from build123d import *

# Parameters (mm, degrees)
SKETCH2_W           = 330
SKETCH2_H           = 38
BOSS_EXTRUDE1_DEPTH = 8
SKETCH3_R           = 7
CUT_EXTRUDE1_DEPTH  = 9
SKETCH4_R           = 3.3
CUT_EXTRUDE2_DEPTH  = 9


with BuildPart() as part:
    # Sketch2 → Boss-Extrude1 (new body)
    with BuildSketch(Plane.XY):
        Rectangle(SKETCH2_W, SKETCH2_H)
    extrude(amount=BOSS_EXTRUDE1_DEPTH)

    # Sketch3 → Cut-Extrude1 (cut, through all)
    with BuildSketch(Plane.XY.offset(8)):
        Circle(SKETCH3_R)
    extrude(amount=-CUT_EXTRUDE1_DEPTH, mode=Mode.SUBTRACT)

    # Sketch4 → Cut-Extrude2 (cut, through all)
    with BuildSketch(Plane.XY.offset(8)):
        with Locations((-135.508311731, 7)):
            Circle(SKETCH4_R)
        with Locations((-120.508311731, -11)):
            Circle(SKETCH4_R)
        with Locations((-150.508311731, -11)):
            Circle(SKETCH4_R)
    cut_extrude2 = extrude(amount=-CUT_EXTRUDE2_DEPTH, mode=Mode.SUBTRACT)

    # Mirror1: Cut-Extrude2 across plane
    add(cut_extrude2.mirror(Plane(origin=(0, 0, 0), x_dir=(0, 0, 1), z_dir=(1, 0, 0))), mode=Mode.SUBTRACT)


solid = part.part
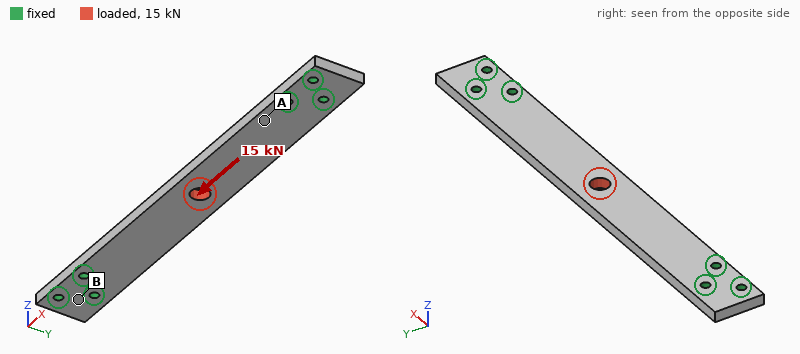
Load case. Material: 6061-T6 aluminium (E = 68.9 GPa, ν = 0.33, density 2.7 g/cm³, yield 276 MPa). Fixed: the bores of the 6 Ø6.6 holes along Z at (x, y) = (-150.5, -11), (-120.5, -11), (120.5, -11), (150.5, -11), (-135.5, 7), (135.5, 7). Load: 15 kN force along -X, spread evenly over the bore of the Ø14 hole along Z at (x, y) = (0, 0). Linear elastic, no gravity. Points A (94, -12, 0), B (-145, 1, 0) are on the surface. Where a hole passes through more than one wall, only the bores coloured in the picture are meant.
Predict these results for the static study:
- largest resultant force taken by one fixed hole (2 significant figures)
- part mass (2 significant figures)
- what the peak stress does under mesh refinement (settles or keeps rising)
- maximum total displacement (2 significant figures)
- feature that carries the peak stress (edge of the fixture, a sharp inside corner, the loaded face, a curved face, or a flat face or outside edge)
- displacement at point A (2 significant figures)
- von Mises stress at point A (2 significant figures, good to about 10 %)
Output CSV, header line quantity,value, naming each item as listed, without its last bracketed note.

quantity,value
largest resultant force taken by one fixed hole,4.1 kN
part mass,260 g
what the peak stress does under mesh refinement,keeps rising
maximum total displacement,49 µm
feature that carries the peak stress,edge of the fixture
displacement at point A,11 µm
von Mises stress at point A,28 MPa
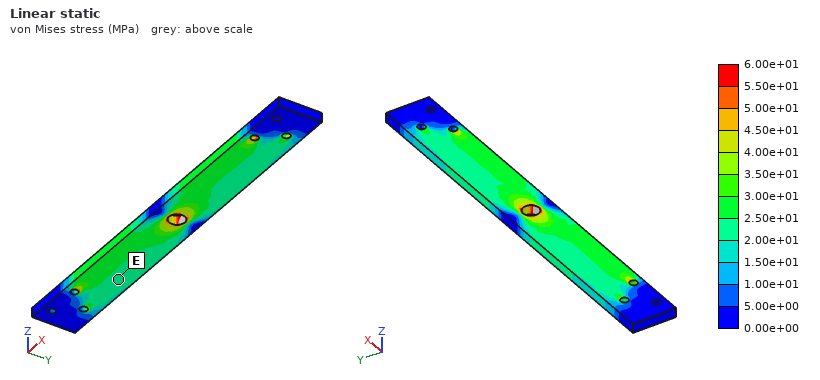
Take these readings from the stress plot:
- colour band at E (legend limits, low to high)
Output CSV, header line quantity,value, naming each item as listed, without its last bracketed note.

quantity,value
colour band at E,2.00e+01 to 2.50e+01 MPa
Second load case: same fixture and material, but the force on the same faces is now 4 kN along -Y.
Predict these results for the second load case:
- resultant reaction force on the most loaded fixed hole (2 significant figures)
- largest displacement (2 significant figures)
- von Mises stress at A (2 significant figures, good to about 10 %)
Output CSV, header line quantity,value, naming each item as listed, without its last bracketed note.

quantity,value
resultant reaction force on the most loaded fixed hole,5.1 kN
largest displacement,0.17 mm
von Mises stress at A,24 MPa
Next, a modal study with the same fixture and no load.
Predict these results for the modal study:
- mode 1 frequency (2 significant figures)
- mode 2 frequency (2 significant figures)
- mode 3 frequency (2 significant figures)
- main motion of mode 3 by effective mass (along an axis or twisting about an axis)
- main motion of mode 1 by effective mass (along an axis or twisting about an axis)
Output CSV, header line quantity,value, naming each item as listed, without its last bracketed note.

quantity,value
mode 1 frequency,690 Hz
mode 2 frequency,1900 Hz
mode 3 frequency,2500 Hz
main motion of mode 3 by effective mass,twisting about X
main motion of mode 1 by effective mass,along Z
